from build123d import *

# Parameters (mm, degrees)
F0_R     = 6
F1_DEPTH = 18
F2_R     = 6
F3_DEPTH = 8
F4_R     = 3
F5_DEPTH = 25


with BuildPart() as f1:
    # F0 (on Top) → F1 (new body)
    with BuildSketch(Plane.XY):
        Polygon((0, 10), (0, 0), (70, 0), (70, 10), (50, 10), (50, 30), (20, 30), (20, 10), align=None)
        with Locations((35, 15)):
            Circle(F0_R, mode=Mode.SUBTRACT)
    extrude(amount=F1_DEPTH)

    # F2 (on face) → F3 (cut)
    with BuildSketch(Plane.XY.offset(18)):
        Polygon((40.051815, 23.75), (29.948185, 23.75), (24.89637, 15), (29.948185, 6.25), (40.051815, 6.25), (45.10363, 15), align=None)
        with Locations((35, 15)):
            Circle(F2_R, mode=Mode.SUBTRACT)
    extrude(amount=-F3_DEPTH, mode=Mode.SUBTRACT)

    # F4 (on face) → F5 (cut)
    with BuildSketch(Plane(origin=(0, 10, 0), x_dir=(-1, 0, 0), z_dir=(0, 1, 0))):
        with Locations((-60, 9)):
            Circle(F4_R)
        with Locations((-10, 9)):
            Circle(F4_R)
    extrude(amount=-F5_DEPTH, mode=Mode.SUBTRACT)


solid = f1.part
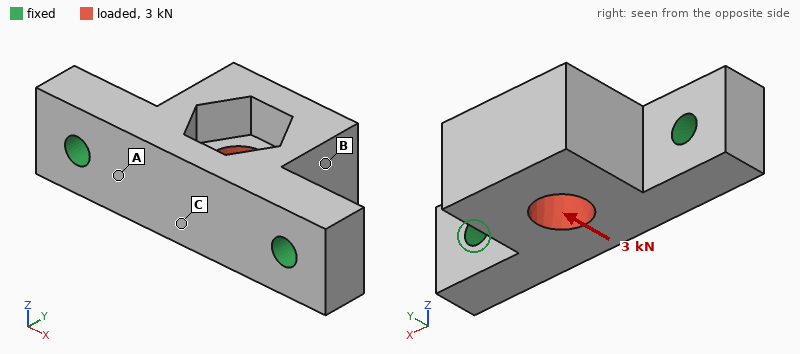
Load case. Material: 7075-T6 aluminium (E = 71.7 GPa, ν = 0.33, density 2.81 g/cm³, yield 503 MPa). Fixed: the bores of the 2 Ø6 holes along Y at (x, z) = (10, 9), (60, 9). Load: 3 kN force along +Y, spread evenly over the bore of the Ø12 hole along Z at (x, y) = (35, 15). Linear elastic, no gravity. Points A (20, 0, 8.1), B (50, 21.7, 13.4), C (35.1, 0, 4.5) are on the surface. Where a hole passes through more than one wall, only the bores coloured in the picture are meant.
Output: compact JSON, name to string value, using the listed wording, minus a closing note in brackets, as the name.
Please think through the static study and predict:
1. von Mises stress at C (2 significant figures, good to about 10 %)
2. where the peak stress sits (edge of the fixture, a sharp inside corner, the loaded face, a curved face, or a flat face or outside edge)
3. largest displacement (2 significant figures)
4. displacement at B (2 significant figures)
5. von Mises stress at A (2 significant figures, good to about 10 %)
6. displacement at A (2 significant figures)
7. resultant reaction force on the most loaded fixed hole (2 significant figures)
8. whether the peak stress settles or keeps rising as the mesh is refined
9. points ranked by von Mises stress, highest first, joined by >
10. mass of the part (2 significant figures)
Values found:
{"von Mises stress at C": "23 MPa", "where the peak stress sits": "edge of the fixture", "largest displacement": "24 µm", "displacement at B": "13 µm", "von Mises stress at A": "13 MPa", "displacement at A": "7.0 µm", "resultant reaction force on the most loaded fixed hole": "1.5 kN", "whether the peak stress settles or keeps rising as the mesh is refined": "keeps rising", "points ranked by von Mises stress, highest first, joined by >": "C > A > B", "mass of the part": "55 g"}
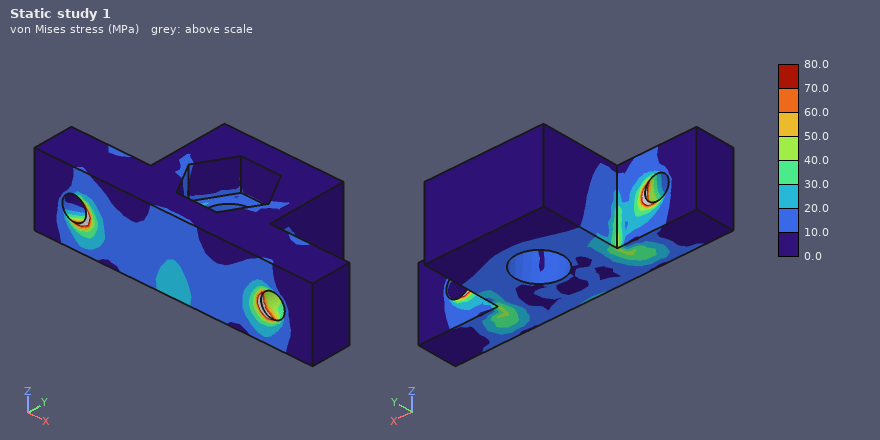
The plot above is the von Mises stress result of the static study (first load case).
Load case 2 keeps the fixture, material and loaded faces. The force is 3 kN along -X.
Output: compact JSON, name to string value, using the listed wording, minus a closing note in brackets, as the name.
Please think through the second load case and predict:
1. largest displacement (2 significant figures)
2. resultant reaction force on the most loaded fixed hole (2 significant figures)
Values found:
{"largest displacement": "12 µm", "resultant reaction force on the most loaded fixed hole": "1.7 kN"}
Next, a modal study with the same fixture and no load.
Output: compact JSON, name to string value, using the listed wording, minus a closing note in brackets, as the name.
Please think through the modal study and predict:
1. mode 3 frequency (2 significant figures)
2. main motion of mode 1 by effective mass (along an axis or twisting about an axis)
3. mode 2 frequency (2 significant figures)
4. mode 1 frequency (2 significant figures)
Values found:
{"mode 3 frequency": "15 kHz", "main motion of mode 1 by effective mass": "along Z", "mode 2 frequency": "14 kHz", "mode 1 frequency": "6900 Hz"}
